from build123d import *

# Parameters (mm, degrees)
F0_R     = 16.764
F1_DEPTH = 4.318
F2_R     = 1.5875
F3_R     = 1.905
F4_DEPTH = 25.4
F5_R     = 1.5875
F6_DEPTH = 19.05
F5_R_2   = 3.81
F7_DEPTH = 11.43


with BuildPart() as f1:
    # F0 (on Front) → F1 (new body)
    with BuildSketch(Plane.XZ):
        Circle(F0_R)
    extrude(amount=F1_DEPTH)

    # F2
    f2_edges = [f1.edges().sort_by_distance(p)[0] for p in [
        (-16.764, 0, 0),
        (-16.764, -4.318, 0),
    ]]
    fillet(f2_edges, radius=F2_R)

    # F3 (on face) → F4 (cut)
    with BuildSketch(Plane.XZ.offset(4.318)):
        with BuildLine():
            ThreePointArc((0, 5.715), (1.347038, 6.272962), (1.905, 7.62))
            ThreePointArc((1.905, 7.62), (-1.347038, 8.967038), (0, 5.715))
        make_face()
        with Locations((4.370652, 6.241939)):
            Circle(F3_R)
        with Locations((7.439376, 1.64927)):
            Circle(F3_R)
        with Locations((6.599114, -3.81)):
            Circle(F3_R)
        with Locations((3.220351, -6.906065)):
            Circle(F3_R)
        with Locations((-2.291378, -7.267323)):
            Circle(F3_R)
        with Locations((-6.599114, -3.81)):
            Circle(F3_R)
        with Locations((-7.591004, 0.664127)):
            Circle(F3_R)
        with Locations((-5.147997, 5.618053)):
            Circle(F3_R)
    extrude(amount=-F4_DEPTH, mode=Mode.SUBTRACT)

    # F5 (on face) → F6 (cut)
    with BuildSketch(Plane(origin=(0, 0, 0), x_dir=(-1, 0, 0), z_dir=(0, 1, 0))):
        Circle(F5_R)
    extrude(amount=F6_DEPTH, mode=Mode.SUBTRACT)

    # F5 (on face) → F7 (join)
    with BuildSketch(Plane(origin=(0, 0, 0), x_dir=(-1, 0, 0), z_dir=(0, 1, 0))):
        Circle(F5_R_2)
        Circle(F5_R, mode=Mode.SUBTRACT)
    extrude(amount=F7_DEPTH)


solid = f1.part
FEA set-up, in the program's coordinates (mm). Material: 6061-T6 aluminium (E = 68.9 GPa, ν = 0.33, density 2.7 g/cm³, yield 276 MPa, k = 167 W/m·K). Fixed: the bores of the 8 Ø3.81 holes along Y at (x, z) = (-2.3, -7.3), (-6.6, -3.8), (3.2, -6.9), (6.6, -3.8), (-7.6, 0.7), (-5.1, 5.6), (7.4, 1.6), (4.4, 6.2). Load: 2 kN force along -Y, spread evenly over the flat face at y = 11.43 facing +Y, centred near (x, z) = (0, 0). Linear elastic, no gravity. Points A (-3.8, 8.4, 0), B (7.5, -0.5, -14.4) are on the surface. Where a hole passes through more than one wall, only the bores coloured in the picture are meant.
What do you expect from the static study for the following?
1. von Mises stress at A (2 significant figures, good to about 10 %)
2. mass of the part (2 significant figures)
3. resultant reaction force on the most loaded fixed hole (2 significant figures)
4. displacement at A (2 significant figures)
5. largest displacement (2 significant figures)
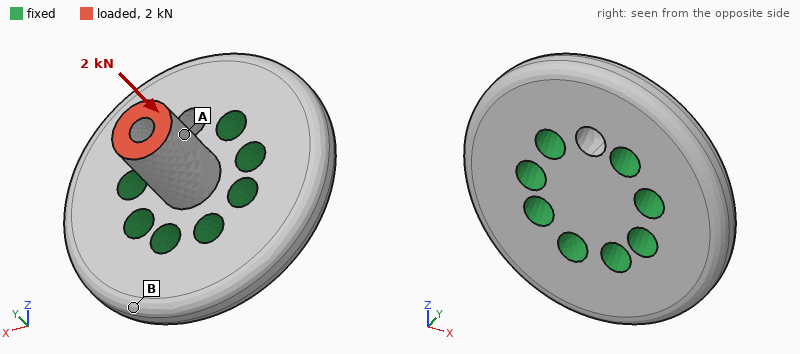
53 MPa
10.0 g
360 N
9.2 µm
12 µm
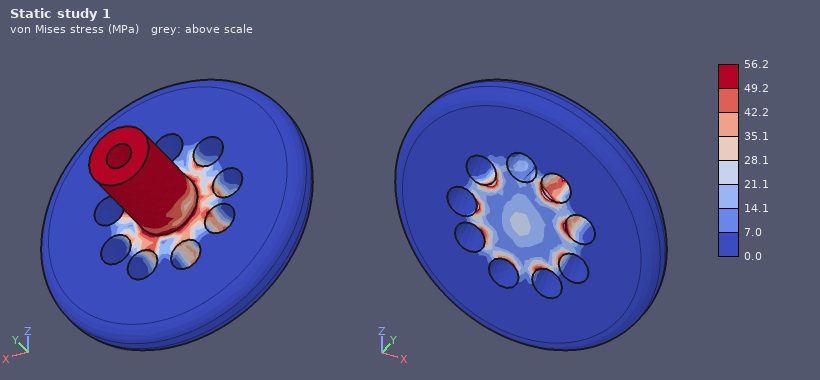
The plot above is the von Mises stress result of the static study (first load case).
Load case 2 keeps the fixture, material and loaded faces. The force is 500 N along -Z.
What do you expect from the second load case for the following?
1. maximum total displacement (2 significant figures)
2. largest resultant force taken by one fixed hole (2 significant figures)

46 µm
360 N
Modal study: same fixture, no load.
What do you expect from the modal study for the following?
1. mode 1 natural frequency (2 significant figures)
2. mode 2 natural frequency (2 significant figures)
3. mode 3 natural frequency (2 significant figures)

28 kHz
29 kHz
38 kHz
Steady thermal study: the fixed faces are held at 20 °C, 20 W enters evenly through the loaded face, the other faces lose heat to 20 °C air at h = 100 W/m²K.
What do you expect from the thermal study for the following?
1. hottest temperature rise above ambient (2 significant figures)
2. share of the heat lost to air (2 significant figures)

41 K
4.6 %
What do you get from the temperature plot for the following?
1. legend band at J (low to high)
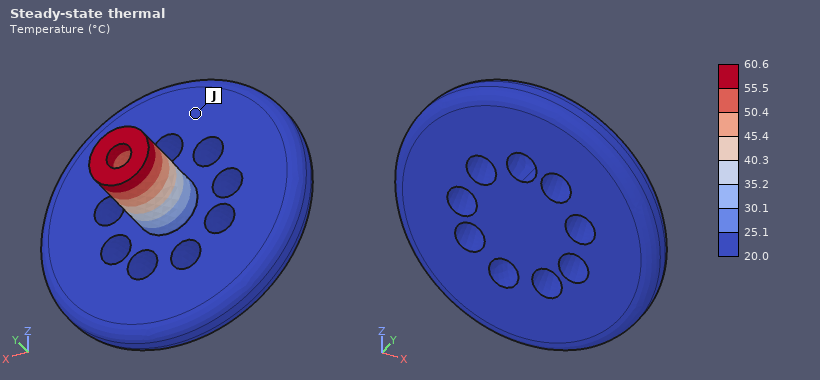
20.0 to 25.1 °C
